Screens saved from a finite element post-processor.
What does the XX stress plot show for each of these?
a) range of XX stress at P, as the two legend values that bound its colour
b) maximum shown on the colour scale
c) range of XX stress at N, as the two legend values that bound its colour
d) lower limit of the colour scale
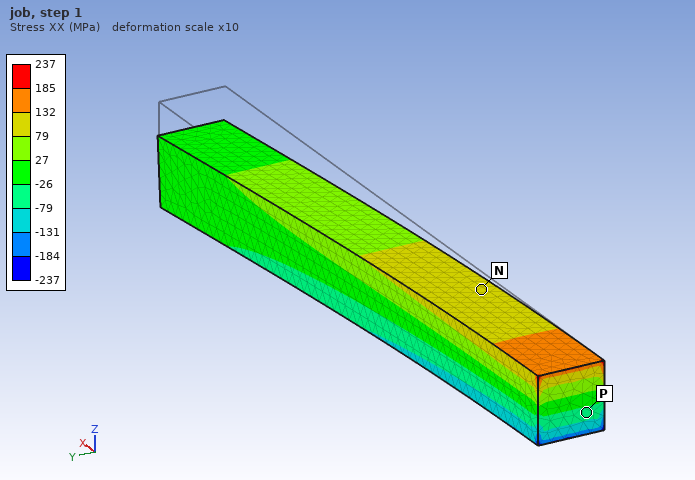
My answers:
-79 to -26 MPa
237 MPa
79 to 132 MPa
-237 MPa
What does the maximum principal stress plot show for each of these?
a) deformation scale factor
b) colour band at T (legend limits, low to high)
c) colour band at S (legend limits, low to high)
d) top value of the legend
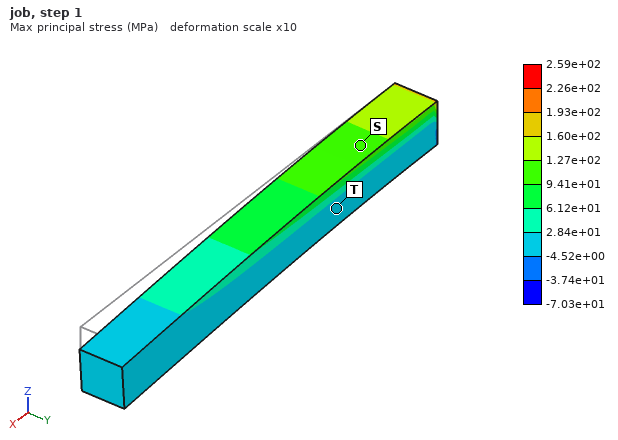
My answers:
10
-4.52e+00 to 2.84e+01 MPa
9.41e+01 to 1.27e+02 MPa
2.59e+02 MPa
